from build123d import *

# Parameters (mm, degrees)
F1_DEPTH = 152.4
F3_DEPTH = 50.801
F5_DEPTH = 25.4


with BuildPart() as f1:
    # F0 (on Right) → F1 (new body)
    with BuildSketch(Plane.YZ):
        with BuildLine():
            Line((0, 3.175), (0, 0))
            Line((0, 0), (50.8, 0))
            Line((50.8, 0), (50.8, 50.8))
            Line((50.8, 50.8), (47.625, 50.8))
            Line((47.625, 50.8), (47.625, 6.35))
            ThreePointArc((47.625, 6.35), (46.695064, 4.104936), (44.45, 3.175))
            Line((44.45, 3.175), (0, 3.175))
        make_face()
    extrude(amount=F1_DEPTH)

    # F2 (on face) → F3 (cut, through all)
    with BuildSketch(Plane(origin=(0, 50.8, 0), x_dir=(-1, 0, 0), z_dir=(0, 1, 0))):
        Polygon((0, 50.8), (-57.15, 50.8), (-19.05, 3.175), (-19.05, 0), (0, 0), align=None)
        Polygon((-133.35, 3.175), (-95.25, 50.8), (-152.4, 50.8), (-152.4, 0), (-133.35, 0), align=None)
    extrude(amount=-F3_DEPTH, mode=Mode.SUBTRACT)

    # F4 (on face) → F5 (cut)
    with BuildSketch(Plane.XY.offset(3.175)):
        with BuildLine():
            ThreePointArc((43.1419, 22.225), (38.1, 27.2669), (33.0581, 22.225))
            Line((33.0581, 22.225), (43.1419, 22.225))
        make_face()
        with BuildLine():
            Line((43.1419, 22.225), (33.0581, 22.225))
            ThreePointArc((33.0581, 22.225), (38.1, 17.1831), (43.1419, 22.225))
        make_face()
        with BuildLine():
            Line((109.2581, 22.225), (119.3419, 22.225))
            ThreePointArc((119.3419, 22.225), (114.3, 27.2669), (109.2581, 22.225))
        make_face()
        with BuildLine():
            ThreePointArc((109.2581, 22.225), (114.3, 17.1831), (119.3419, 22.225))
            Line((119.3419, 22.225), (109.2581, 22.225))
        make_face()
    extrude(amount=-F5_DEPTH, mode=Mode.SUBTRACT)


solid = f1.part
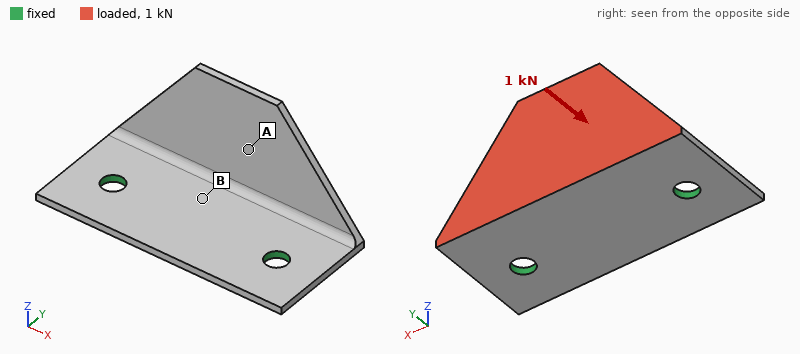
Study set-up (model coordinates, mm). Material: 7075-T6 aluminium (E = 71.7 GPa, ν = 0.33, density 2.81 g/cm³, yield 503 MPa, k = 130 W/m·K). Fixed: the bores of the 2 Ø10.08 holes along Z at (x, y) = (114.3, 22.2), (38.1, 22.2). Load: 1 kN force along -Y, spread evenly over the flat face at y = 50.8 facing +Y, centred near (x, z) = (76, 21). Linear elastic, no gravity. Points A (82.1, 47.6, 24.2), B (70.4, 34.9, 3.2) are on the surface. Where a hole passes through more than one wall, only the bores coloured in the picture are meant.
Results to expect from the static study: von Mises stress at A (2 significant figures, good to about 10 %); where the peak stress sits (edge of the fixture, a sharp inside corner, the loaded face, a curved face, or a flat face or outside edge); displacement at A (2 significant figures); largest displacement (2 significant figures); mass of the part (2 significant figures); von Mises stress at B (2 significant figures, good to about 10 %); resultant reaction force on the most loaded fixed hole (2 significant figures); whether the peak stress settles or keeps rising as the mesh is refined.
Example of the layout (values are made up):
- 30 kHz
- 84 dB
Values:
- 33 MPa
- edge of the fixture
- 0.67 mm
- 1.6 mm
- 83 g
- 78 MPa
- 510 N
- keeps rising
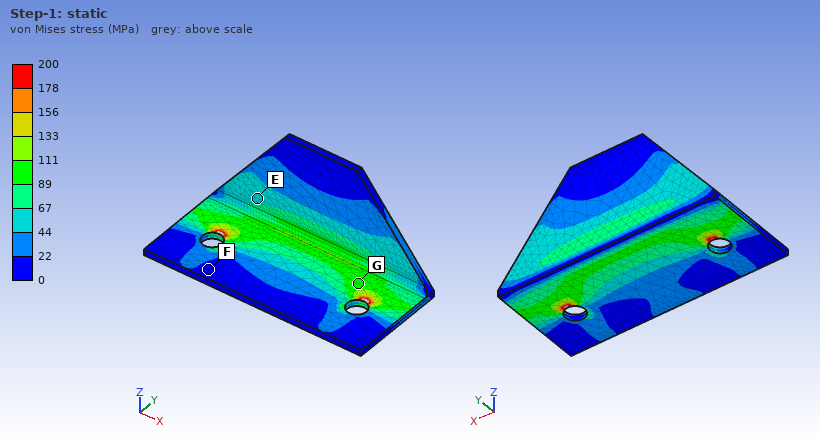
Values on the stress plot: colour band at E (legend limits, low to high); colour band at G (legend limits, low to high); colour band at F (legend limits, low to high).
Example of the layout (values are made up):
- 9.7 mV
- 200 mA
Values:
- 44 to 67 MPa
- 89 to 111 MPa
- 0 to 22 MPa
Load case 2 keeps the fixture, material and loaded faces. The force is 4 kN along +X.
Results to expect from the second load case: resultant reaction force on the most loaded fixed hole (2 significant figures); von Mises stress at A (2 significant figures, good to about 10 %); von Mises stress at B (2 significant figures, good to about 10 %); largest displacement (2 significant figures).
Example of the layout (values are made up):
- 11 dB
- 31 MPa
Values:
- 2.6 kN
- 37 MPa
- 69 MPa
- 0.52 mm
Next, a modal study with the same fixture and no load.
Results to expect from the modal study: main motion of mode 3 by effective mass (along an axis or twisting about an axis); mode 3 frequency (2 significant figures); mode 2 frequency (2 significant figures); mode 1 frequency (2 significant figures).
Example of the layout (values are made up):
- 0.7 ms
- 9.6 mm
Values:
- along Z
- 2100 Hz
- 1800 Hz
- 810 Hz
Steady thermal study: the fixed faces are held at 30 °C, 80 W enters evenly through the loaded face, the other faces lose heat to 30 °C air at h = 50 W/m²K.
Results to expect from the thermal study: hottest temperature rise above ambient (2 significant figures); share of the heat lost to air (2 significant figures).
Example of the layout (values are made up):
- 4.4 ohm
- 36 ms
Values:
- 79 K
- 29 %
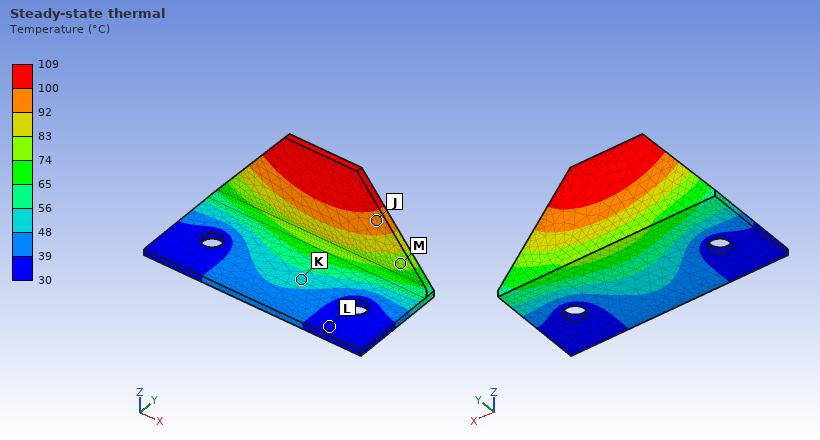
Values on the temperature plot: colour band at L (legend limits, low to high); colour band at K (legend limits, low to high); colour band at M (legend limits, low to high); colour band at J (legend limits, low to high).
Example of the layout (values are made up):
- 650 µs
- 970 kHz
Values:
- 30 to 39 °C
- 48 to 56 °C
- 74 to 83 °C
- 92 to 100 °C
